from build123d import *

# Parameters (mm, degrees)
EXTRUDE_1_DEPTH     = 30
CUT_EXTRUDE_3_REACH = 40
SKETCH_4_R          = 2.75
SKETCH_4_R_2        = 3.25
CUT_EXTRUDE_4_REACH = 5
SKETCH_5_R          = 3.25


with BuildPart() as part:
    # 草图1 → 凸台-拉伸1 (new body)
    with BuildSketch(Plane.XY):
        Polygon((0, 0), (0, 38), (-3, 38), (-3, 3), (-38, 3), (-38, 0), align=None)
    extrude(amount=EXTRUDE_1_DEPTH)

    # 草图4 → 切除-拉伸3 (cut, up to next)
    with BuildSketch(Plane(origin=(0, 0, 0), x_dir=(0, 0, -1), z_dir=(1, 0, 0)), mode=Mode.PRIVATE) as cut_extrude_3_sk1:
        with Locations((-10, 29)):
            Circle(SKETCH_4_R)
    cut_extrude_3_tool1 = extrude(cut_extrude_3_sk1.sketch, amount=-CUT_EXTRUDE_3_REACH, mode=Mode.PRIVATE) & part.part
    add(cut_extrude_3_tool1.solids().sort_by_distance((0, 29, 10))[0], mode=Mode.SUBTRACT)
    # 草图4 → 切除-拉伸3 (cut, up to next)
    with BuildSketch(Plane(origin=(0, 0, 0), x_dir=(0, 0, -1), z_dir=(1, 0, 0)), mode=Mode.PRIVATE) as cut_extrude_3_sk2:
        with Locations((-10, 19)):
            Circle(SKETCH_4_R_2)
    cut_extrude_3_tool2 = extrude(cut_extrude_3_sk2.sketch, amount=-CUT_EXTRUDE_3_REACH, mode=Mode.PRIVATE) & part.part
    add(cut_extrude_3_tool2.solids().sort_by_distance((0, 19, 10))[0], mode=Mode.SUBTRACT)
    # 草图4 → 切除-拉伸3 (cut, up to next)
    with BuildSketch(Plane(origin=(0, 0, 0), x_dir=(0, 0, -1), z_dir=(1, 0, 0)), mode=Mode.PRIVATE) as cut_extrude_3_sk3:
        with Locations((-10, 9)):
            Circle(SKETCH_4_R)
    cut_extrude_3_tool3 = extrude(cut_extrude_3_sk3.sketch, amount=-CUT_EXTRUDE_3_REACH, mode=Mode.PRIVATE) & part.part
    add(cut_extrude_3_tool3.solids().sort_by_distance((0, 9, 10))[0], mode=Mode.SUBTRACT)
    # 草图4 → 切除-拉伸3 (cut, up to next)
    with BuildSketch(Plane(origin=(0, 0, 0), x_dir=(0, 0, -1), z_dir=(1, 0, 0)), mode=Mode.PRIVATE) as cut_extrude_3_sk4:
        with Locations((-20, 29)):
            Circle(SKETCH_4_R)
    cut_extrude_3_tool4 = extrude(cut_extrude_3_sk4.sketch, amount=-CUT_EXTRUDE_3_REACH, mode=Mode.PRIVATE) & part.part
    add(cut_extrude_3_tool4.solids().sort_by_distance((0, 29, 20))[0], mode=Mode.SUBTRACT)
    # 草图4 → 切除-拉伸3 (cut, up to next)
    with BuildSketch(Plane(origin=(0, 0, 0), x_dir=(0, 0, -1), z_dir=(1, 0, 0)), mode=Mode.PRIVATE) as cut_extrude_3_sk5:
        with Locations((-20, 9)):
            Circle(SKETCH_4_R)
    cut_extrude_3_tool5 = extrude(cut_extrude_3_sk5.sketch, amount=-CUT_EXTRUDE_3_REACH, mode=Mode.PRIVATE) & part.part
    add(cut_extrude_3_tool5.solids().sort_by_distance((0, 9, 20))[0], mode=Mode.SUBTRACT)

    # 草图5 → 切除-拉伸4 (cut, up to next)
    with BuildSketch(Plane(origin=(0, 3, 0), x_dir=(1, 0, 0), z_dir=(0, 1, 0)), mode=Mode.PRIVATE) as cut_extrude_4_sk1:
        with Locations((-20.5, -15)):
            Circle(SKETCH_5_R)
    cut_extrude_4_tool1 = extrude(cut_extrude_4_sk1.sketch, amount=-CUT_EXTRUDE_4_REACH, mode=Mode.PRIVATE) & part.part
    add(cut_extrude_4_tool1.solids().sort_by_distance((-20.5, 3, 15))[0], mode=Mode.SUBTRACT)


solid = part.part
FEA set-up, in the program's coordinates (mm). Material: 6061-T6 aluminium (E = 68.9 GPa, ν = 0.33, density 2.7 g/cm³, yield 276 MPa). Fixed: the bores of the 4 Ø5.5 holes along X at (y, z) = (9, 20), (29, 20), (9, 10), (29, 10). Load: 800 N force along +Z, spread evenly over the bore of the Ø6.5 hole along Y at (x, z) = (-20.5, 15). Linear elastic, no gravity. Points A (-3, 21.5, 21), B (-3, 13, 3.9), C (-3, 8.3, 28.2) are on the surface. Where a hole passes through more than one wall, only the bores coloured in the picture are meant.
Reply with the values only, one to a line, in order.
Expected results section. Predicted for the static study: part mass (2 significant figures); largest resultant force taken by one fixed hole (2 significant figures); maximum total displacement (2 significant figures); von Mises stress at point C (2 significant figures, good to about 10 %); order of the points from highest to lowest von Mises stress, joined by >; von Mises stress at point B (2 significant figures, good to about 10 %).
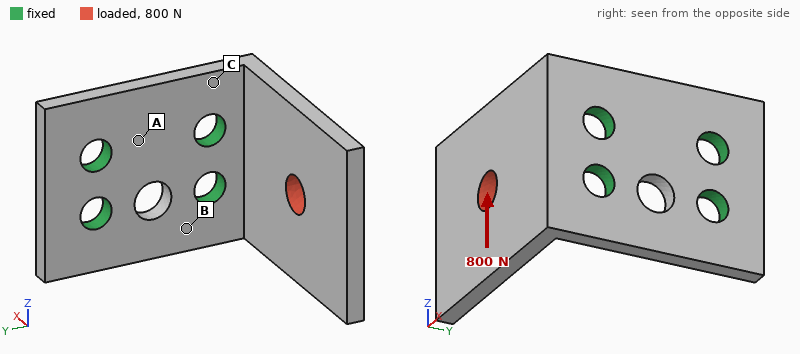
16 g
1.1 kN
0.17 mm
69 MPa
C > B > A
36 MPa
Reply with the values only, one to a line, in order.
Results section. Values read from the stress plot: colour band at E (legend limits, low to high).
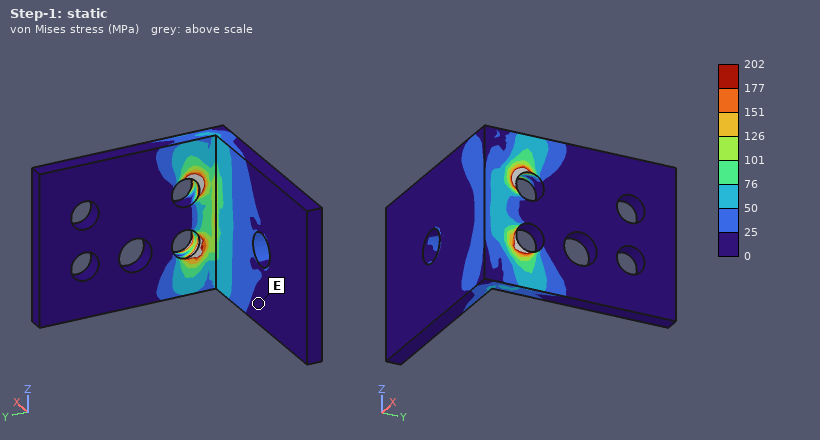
0 to 25 MPa
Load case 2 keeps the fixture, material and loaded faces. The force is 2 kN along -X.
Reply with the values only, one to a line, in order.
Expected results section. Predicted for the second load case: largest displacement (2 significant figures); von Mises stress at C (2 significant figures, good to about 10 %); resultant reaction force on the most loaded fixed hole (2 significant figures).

0.29 mm
70 MPa
1.0 kN
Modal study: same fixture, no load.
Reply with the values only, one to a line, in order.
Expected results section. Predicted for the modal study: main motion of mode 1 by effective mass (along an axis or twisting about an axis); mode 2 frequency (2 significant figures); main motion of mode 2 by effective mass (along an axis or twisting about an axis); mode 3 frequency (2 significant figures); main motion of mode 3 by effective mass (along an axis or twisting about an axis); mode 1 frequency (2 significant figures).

along Y
4100 Hz
along Z
5300 Hz
along Z
1500 Hz
